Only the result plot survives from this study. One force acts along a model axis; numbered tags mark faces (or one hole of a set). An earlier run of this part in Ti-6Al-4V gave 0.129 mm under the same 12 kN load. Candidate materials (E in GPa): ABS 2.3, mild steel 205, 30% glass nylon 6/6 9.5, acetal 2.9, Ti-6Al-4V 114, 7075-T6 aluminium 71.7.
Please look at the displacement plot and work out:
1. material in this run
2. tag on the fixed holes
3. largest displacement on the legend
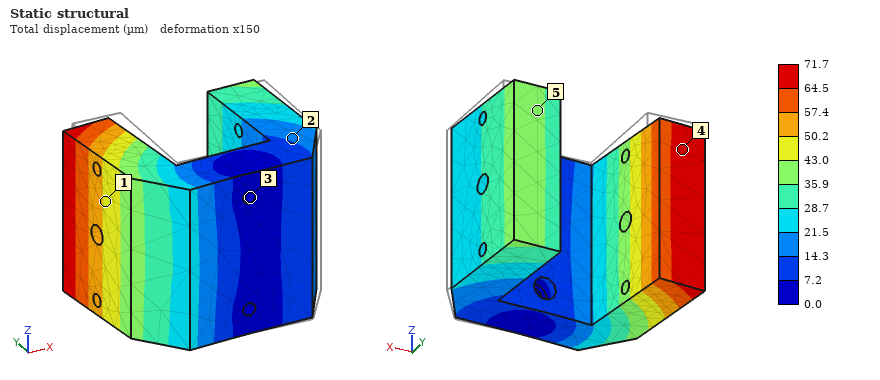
mild steel
3
71.7 µm
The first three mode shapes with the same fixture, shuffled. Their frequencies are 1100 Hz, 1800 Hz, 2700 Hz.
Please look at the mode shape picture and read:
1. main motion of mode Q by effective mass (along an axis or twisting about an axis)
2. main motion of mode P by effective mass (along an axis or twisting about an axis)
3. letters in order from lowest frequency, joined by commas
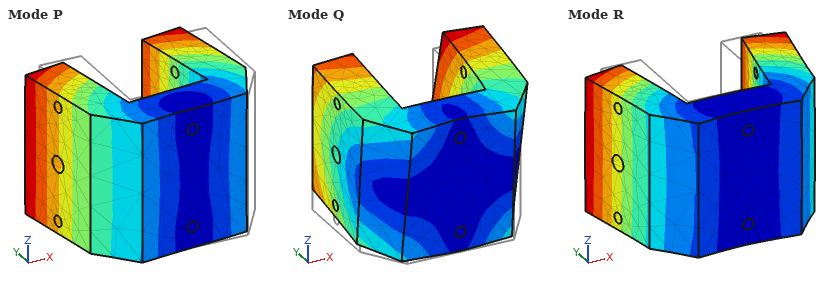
along Z
along X
P, R, Q
